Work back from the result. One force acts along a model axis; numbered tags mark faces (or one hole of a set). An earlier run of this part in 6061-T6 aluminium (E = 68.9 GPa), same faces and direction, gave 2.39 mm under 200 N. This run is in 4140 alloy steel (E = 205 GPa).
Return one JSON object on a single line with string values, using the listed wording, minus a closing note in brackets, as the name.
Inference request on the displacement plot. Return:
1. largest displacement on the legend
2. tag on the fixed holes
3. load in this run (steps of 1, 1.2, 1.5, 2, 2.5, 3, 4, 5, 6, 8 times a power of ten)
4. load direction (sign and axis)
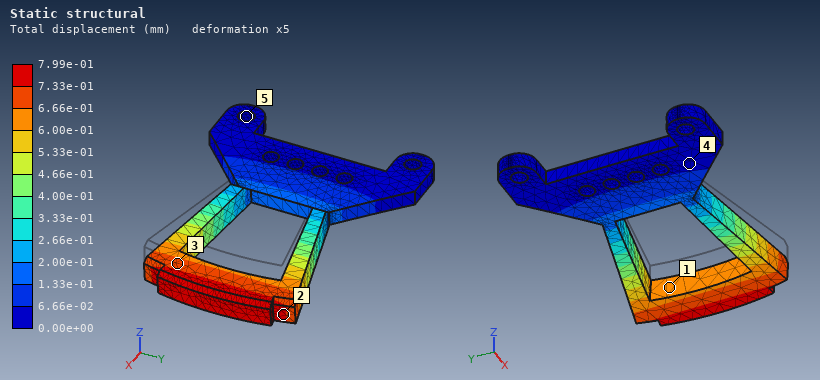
{"largest displacement on the legend": "7.99e-01 mm", "tag on the fixed holes": "5", "load in this run": "200 N", "load direction": "-Z"}
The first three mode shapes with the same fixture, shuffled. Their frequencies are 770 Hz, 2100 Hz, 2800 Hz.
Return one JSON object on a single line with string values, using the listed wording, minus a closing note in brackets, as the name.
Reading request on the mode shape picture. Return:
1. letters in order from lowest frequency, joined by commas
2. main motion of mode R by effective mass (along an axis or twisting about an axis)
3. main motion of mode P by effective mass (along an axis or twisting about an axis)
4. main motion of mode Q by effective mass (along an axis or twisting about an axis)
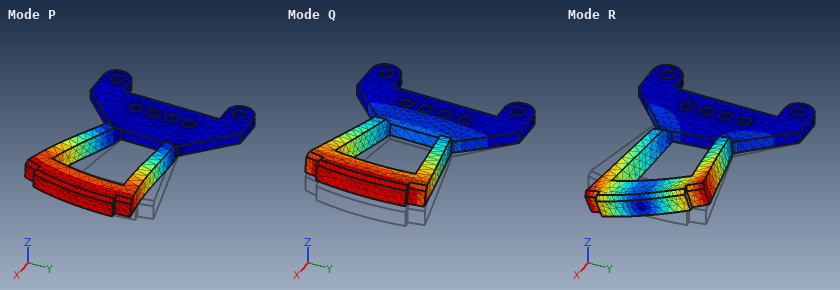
{"letters in order from lowest frequency, joined by commas": "Q, P, R", "main motion of mode R by effective mass": "twisting about X", "main motion of mode P by effective mass": "along Y", "main motion of mode Q by effective mass": "along Z"}
